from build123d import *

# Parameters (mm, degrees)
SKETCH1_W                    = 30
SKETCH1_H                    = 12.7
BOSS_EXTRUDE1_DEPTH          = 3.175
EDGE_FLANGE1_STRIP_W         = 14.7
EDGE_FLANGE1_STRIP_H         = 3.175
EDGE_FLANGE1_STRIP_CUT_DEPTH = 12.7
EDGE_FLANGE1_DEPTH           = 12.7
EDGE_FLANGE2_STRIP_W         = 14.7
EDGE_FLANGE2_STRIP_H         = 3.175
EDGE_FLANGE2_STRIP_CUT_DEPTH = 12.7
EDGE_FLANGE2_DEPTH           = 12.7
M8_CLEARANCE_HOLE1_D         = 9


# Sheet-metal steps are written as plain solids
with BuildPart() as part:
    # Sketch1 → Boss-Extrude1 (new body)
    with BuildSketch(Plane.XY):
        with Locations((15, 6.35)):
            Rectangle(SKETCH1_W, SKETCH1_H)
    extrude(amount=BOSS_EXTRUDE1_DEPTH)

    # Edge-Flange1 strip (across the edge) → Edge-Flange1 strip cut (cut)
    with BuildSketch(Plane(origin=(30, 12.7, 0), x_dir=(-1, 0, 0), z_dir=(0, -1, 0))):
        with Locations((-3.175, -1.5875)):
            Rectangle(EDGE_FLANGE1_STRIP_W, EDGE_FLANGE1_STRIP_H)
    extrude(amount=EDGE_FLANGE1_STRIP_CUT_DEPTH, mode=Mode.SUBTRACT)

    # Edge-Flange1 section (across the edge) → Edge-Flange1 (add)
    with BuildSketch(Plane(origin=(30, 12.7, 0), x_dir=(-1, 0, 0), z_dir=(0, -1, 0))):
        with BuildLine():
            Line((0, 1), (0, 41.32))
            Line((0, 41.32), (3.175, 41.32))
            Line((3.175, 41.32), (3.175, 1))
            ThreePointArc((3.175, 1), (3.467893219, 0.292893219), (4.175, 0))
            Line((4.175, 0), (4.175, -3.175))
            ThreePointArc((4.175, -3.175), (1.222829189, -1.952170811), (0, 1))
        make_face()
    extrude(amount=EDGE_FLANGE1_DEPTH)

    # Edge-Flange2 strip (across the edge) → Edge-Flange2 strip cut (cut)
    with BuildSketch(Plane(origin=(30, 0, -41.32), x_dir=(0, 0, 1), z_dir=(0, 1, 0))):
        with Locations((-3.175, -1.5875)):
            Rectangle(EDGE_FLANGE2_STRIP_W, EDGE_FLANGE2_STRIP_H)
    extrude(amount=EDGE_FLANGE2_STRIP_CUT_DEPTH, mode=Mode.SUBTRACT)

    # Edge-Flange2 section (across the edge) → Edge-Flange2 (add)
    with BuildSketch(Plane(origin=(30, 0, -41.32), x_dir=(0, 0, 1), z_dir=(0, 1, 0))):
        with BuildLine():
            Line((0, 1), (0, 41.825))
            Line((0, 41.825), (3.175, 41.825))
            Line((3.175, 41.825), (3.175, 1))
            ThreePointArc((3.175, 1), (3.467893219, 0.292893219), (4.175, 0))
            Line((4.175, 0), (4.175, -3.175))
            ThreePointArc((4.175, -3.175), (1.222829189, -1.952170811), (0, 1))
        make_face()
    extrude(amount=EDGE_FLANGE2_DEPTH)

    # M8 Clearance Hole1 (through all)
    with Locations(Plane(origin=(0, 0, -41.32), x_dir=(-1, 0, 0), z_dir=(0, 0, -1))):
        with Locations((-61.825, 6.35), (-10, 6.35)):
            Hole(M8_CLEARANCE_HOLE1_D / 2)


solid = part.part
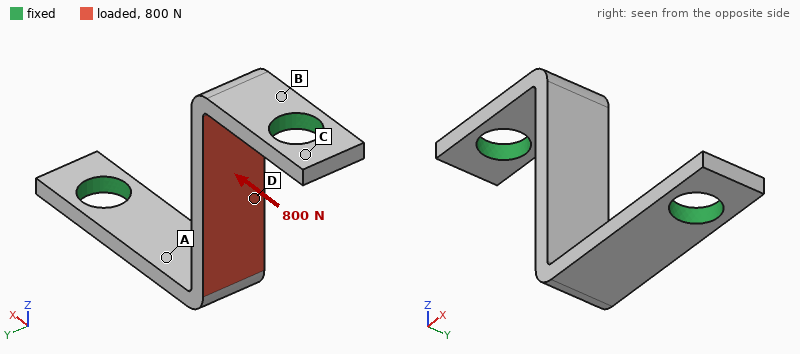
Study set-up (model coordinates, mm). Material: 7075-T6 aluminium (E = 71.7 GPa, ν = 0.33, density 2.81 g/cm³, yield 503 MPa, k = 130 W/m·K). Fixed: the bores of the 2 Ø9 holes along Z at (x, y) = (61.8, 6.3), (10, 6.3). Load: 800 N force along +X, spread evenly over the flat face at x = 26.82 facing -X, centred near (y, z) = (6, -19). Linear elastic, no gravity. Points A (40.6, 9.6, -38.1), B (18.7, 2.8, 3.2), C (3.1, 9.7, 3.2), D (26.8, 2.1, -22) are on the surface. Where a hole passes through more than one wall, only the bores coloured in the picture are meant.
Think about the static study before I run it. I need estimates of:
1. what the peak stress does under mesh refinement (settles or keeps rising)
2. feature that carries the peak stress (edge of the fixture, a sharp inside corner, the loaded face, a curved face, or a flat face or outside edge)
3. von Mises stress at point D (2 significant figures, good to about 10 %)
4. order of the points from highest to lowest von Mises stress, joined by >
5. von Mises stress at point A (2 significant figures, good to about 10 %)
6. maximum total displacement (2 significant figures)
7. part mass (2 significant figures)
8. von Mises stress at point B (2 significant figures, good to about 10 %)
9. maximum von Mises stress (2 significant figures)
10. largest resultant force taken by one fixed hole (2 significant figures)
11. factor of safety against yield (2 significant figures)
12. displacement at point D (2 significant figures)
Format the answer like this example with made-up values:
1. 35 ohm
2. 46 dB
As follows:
1. settles
2. a curved face
3. 130 MPa
4. D > B > A > C
5. 63 MPa
6. 0.21 mm
7. 11 g
8. 93 MPa
9. 160 MPa
10. 420 N
11. 3.2
12. 0.21 mm
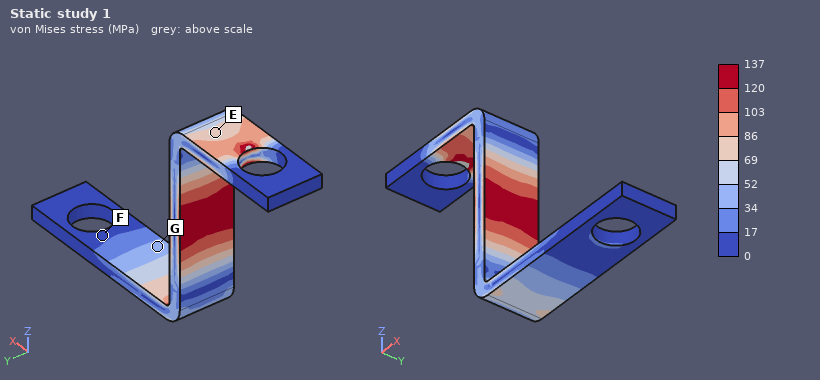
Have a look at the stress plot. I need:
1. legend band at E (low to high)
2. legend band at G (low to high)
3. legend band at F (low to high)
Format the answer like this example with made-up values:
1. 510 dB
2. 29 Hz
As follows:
1. 69 to 86 MPa
2. 34 to 52 MPa
3. 0 to 17 MPa
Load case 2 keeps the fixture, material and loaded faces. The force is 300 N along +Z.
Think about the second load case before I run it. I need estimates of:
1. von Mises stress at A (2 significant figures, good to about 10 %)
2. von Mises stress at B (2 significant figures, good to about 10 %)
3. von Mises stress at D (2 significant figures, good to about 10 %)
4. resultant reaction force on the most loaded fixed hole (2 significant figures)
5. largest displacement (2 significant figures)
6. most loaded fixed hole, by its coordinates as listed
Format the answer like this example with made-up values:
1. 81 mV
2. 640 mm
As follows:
1. 10 MPa
2. 70 MPa
3. 26 MPa
4. 270 N
5. 90 µm
6. (10, 6.3)
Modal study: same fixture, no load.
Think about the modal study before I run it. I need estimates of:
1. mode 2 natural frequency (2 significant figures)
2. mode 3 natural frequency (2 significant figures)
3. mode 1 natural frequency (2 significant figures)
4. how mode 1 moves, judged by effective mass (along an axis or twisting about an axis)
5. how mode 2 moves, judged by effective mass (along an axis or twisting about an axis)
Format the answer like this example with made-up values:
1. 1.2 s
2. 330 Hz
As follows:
1. 5900 Hz
2. 7700 Hz
3. 3800 Hz
4. along Z
5. along Y
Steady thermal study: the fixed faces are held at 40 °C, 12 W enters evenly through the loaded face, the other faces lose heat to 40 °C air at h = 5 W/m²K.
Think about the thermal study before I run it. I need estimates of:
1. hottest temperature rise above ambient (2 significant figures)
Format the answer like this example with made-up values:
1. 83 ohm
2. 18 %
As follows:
1. 36 K
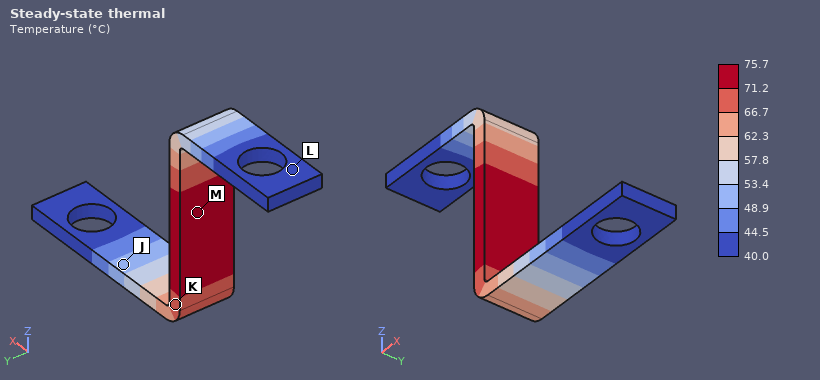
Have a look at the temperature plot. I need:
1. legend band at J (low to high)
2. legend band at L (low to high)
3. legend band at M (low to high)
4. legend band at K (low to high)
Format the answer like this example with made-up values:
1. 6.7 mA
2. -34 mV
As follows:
1. 48.9 to 53.4 °C
2. 40.0 to 44.5 °C
3. 71.2 to 75.7 °C
4. 66.7 to 71.2 °C
